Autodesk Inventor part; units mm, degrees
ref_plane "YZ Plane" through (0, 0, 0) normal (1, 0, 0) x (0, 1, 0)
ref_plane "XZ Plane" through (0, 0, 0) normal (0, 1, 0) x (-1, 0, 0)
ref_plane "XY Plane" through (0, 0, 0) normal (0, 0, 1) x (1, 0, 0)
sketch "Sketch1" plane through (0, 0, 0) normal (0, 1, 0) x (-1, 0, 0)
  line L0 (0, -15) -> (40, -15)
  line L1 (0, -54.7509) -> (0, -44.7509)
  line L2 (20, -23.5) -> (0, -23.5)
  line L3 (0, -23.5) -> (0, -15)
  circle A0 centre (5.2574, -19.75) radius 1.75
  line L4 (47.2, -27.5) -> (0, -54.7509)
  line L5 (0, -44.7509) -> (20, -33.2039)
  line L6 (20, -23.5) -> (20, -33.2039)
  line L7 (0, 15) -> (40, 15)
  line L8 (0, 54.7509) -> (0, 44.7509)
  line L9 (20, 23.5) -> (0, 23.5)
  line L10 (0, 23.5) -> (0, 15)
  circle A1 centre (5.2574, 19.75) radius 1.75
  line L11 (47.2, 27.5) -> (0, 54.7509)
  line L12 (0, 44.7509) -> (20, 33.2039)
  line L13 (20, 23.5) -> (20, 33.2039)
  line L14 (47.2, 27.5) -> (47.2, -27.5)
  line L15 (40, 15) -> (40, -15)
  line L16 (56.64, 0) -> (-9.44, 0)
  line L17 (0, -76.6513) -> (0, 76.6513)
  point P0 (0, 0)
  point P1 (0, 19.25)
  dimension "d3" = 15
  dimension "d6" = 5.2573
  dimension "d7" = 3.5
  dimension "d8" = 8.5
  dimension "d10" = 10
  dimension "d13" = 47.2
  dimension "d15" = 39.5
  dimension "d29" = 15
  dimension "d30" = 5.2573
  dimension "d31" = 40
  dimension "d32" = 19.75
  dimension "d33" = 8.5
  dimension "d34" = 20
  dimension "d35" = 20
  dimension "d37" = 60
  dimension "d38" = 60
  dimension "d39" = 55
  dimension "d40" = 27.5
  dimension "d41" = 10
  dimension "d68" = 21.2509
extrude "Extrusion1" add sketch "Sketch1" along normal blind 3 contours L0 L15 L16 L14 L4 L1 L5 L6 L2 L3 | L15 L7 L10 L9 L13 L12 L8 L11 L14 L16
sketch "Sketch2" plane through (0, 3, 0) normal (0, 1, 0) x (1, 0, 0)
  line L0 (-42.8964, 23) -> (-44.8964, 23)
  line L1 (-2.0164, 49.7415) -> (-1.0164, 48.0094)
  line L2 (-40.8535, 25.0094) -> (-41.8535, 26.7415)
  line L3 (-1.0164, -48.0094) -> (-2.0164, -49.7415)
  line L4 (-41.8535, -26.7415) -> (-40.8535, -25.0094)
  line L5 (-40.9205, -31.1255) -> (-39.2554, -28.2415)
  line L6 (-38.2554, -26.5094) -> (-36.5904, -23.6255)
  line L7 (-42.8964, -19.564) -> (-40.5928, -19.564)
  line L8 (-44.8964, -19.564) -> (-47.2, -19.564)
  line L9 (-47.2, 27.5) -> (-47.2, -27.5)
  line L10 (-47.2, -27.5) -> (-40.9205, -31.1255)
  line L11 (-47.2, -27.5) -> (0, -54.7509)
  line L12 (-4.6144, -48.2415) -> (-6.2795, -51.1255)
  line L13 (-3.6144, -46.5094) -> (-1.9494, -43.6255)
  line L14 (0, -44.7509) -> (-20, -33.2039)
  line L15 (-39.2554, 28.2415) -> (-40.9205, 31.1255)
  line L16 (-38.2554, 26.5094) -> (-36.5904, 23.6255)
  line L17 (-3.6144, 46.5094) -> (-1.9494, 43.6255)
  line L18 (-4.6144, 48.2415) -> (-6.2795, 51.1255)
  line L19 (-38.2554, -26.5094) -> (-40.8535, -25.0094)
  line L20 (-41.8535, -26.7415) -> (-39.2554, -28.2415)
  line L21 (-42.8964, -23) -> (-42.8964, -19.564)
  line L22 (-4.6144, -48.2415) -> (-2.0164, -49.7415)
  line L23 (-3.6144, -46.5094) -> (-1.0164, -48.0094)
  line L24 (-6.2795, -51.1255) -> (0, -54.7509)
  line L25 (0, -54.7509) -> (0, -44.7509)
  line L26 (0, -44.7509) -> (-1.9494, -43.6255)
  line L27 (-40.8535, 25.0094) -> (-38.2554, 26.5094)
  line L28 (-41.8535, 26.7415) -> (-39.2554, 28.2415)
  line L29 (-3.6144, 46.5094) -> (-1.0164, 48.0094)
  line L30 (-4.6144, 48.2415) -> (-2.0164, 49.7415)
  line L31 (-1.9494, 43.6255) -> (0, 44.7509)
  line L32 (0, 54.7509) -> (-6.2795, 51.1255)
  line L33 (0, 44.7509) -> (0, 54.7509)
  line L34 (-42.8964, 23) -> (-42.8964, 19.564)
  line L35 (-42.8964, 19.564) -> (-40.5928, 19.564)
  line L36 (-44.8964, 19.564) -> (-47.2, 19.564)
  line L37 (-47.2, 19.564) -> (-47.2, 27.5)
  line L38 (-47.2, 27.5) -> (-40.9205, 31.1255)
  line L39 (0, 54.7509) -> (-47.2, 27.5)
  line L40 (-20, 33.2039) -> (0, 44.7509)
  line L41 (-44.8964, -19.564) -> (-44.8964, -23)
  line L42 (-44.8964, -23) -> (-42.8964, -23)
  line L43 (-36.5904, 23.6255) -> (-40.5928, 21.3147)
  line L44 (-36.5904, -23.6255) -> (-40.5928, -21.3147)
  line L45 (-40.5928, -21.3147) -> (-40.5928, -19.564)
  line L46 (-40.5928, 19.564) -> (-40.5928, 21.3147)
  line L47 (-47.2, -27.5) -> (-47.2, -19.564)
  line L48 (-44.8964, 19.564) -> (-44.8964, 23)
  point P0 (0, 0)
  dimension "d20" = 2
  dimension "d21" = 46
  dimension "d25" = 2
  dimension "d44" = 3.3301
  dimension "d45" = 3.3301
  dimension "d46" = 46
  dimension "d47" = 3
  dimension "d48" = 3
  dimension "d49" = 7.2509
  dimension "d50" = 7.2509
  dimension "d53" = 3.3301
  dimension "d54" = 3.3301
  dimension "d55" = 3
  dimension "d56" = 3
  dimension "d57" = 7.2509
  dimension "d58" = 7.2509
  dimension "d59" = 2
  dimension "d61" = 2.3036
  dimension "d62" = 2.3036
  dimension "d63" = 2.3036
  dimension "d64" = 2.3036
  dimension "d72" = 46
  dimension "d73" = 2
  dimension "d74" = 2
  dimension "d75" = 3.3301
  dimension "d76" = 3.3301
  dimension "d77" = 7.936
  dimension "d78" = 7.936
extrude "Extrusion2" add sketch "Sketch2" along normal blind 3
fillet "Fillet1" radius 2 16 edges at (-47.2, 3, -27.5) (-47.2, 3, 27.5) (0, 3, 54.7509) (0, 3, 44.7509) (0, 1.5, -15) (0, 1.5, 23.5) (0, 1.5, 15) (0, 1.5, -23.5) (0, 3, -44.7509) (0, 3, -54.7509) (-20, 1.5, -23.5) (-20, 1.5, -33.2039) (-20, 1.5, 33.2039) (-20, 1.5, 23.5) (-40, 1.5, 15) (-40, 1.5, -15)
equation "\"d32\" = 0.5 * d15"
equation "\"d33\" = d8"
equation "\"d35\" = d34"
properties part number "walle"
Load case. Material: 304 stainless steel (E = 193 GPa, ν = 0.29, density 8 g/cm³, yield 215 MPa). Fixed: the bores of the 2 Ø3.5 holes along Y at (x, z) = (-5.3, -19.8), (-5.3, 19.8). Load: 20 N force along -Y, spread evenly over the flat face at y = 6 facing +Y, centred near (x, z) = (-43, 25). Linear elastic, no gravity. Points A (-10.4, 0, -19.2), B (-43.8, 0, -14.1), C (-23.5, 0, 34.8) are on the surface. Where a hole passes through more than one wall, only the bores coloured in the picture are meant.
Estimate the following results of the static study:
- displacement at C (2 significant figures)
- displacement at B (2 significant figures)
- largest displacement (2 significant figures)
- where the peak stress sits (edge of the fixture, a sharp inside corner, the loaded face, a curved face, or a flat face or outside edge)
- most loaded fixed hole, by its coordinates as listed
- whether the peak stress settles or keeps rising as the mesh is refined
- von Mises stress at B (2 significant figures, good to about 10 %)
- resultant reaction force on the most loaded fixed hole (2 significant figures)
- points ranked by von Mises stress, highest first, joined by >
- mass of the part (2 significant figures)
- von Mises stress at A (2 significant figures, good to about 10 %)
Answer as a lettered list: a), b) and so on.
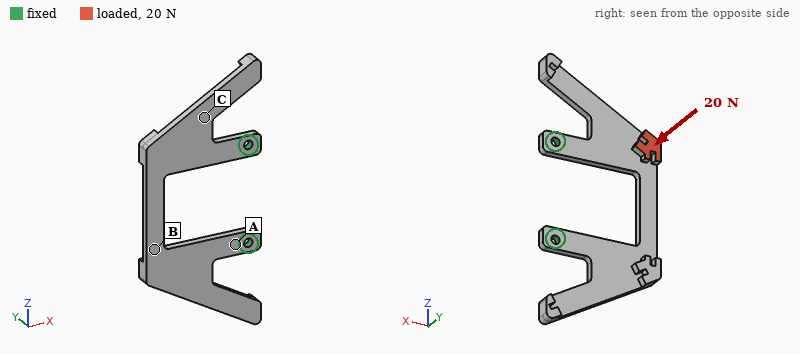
a) 26 µm
b) 31 µm
c) 68 µm
d) edge of the fixture
e) (-5.3, 19.8)
f) keeps rising
g) 10 MPa
h) 17 N
i) A > B > C
j) 54 g
k) 16 MPa
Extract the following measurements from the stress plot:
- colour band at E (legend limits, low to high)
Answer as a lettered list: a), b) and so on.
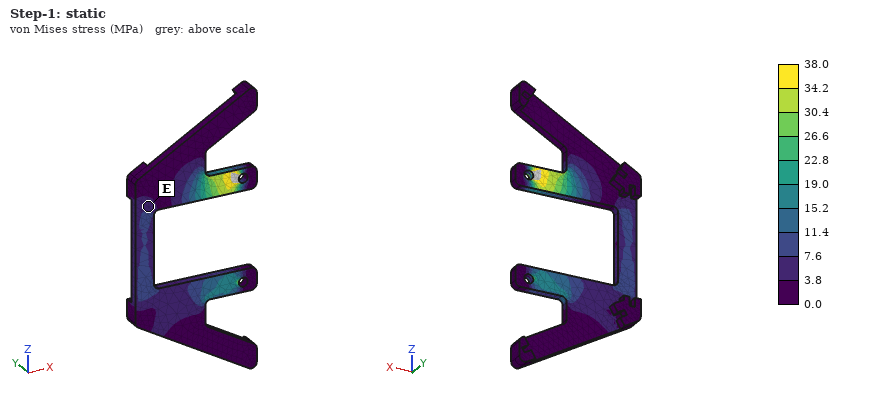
a) 3.8 to 7.6 MPa
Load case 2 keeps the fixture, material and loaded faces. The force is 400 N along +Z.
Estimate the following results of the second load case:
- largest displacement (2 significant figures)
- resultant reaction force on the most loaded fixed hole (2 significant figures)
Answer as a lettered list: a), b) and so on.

a) 0.13 mm
b) 280 N
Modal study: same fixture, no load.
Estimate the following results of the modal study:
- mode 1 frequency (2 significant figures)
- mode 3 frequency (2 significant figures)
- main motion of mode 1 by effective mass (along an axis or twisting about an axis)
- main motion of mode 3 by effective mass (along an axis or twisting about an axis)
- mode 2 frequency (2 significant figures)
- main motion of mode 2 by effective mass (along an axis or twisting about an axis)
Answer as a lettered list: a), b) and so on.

a) 760 Hz
b) 1100 Hz
c) along Y
d) along Y
e) 1000 Hz
f) twisting about X
